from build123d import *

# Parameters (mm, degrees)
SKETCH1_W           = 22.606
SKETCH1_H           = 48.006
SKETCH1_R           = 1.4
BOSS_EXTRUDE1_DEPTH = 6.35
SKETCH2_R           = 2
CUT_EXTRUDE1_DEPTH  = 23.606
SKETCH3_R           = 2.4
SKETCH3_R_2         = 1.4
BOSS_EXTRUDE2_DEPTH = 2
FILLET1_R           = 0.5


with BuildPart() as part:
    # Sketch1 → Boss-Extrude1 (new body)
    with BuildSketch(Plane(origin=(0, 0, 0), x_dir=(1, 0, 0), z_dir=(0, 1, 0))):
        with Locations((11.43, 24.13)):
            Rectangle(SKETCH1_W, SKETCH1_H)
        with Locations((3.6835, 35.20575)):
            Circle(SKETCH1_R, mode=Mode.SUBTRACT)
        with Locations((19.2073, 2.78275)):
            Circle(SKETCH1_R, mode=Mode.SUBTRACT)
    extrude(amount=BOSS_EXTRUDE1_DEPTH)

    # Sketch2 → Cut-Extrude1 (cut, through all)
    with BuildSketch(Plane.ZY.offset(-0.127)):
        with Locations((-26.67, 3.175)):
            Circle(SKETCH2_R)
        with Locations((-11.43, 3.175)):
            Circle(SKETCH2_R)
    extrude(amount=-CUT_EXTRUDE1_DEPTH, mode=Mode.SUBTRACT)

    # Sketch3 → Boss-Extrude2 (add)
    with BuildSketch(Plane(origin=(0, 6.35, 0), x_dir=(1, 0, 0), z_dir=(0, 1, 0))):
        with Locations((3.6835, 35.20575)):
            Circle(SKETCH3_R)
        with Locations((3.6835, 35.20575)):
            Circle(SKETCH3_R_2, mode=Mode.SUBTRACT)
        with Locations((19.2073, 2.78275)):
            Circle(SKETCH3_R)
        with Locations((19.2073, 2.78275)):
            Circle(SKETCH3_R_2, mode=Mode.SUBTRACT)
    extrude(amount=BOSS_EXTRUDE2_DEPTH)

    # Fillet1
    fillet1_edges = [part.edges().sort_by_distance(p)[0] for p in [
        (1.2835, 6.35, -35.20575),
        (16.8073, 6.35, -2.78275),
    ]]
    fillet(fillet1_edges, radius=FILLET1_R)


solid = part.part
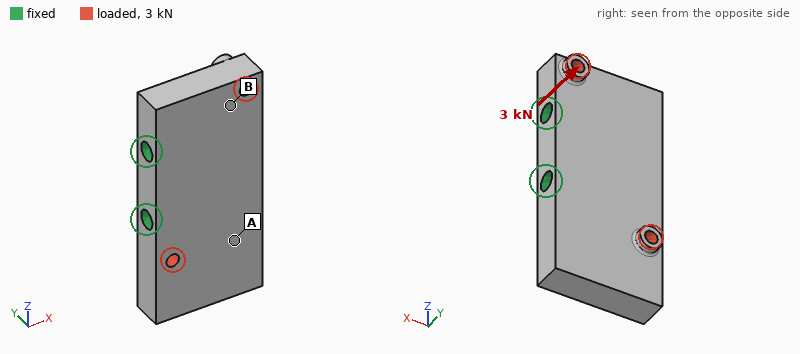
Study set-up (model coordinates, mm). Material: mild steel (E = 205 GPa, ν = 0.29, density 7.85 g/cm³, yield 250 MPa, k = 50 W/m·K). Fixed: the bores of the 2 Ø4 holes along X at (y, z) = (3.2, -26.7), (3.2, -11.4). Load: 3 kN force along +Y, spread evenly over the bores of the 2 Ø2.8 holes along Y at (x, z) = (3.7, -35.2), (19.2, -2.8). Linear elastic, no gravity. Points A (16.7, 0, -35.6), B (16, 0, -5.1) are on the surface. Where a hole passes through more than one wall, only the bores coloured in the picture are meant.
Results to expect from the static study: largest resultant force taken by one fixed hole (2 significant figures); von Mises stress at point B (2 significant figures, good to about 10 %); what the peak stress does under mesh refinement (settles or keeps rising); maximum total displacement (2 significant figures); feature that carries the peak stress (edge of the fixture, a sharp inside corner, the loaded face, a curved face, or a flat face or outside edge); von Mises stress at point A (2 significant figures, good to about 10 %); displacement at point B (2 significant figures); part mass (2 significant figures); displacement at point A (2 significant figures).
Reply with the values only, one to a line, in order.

1.5 kN
59 MPa
keeps rising
15 µm
edge of the fixture
26 MPa
4.1 µm
49 g
2.4 µm
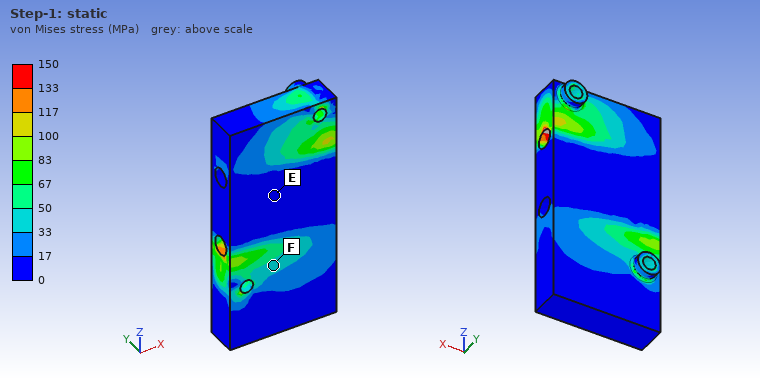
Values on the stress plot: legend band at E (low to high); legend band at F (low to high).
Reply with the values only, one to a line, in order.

0 to 17 MPa
33 to 50 MPa
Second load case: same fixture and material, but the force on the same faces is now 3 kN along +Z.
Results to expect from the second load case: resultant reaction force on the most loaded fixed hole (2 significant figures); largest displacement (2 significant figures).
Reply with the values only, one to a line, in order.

1.5 kN
4.3 µm
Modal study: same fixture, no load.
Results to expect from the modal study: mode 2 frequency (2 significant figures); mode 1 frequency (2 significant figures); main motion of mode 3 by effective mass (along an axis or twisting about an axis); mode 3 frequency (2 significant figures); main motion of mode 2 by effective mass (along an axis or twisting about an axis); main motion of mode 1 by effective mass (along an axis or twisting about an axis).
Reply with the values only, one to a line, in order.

23 kHz
11 kHz
along X
27 kHz
twisting about Z
along Y
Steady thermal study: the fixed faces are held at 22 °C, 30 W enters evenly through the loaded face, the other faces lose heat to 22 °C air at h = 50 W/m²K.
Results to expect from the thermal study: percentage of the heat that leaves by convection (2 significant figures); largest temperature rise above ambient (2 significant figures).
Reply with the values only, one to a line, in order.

4.2 %
44 K
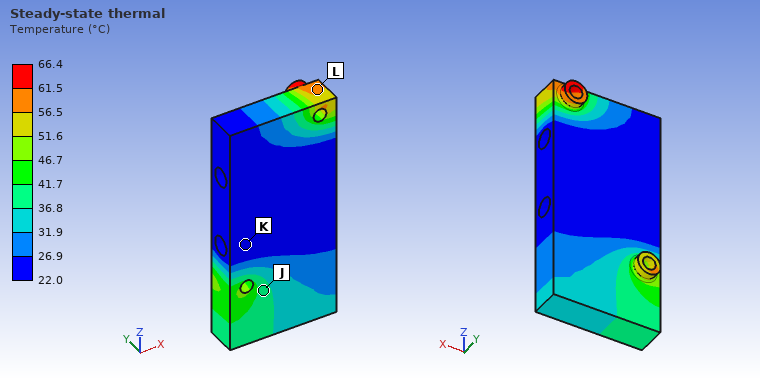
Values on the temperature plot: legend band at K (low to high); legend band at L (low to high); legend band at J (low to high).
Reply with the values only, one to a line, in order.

22.0 to 26.9 °C
56.5 to 61.5 °C
36.8 to 41.7 °C
